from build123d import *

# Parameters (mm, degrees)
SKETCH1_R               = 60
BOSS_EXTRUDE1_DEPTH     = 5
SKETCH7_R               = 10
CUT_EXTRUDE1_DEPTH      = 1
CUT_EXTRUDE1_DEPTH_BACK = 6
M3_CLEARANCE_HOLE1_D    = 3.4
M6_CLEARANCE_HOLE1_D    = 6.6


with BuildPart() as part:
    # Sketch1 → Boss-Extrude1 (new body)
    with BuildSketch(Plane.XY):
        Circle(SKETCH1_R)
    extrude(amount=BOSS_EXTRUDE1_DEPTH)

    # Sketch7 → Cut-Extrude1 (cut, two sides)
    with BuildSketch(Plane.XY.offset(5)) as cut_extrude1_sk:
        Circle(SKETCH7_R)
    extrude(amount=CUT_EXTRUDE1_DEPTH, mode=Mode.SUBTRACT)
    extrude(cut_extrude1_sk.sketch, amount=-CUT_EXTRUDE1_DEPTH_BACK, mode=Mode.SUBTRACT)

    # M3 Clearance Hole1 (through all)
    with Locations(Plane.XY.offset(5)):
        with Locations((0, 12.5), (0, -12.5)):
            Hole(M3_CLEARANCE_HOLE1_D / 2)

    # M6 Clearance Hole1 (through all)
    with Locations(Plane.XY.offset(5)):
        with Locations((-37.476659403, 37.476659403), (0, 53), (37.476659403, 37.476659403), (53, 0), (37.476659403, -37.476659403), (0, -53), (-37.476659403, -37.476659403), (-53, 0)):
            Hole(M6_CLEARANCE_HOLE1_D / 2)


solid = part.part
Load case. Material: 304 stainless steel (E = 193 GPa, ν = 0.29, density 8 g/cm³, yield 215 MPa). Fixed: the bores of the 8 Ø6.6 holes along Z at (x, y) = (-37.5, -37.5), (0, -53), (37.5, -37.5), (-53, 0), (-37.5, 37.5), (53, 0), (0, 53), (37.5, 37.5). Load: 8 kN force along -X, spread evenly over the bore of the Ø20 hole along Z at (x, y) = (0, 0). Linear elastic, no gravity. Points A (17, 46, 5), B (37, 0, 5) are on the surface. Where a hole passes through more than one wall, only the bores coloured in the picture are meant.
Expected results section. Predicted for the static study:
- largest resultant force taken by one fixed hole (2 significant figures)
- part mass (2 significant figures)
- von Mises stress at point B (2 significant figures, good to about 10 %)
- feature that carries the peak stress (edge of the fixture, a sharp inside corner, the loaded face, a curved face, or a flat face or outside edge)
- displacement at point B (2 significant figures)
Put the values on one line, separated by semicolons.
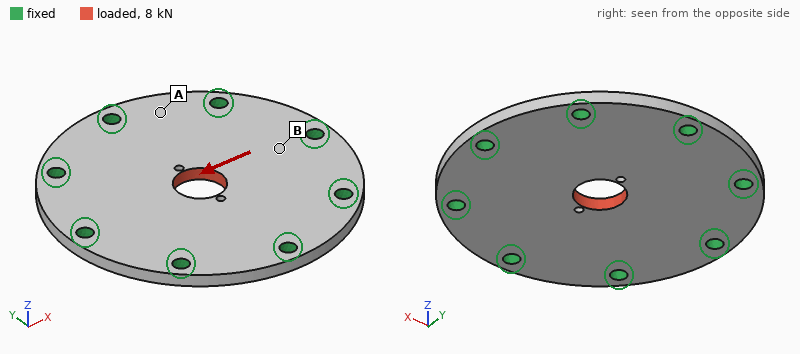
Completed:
1.7 kN; 430 g; 17 MPa; a curved face; 1.4 µm
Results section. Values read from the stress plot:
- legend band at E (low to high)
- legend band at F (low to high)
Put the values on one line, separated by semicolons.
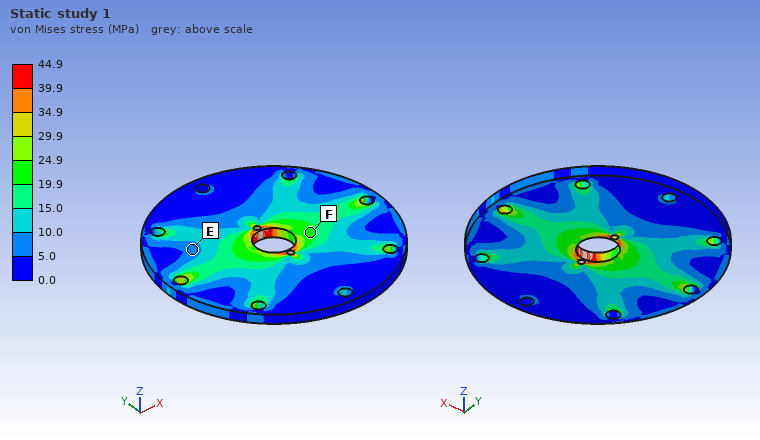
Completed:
5.0 to 10.0 MPa; 19.9 to 24.9 MPa
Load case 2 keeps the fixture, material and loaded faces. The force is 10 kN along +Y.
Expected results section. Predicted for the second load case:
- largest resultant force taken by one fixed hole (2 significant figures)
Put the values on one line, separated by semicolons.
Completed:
2.0 kN
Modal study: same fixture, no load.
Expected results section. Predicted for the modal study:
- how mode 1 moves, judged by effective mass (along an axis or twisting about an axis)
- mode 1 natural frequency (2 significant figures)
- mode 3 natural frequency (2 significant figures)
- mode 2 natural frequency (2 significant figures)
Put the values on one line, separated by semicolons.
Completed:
along Z; 4000 Hz; 7700 Hz; 7700 Hz
